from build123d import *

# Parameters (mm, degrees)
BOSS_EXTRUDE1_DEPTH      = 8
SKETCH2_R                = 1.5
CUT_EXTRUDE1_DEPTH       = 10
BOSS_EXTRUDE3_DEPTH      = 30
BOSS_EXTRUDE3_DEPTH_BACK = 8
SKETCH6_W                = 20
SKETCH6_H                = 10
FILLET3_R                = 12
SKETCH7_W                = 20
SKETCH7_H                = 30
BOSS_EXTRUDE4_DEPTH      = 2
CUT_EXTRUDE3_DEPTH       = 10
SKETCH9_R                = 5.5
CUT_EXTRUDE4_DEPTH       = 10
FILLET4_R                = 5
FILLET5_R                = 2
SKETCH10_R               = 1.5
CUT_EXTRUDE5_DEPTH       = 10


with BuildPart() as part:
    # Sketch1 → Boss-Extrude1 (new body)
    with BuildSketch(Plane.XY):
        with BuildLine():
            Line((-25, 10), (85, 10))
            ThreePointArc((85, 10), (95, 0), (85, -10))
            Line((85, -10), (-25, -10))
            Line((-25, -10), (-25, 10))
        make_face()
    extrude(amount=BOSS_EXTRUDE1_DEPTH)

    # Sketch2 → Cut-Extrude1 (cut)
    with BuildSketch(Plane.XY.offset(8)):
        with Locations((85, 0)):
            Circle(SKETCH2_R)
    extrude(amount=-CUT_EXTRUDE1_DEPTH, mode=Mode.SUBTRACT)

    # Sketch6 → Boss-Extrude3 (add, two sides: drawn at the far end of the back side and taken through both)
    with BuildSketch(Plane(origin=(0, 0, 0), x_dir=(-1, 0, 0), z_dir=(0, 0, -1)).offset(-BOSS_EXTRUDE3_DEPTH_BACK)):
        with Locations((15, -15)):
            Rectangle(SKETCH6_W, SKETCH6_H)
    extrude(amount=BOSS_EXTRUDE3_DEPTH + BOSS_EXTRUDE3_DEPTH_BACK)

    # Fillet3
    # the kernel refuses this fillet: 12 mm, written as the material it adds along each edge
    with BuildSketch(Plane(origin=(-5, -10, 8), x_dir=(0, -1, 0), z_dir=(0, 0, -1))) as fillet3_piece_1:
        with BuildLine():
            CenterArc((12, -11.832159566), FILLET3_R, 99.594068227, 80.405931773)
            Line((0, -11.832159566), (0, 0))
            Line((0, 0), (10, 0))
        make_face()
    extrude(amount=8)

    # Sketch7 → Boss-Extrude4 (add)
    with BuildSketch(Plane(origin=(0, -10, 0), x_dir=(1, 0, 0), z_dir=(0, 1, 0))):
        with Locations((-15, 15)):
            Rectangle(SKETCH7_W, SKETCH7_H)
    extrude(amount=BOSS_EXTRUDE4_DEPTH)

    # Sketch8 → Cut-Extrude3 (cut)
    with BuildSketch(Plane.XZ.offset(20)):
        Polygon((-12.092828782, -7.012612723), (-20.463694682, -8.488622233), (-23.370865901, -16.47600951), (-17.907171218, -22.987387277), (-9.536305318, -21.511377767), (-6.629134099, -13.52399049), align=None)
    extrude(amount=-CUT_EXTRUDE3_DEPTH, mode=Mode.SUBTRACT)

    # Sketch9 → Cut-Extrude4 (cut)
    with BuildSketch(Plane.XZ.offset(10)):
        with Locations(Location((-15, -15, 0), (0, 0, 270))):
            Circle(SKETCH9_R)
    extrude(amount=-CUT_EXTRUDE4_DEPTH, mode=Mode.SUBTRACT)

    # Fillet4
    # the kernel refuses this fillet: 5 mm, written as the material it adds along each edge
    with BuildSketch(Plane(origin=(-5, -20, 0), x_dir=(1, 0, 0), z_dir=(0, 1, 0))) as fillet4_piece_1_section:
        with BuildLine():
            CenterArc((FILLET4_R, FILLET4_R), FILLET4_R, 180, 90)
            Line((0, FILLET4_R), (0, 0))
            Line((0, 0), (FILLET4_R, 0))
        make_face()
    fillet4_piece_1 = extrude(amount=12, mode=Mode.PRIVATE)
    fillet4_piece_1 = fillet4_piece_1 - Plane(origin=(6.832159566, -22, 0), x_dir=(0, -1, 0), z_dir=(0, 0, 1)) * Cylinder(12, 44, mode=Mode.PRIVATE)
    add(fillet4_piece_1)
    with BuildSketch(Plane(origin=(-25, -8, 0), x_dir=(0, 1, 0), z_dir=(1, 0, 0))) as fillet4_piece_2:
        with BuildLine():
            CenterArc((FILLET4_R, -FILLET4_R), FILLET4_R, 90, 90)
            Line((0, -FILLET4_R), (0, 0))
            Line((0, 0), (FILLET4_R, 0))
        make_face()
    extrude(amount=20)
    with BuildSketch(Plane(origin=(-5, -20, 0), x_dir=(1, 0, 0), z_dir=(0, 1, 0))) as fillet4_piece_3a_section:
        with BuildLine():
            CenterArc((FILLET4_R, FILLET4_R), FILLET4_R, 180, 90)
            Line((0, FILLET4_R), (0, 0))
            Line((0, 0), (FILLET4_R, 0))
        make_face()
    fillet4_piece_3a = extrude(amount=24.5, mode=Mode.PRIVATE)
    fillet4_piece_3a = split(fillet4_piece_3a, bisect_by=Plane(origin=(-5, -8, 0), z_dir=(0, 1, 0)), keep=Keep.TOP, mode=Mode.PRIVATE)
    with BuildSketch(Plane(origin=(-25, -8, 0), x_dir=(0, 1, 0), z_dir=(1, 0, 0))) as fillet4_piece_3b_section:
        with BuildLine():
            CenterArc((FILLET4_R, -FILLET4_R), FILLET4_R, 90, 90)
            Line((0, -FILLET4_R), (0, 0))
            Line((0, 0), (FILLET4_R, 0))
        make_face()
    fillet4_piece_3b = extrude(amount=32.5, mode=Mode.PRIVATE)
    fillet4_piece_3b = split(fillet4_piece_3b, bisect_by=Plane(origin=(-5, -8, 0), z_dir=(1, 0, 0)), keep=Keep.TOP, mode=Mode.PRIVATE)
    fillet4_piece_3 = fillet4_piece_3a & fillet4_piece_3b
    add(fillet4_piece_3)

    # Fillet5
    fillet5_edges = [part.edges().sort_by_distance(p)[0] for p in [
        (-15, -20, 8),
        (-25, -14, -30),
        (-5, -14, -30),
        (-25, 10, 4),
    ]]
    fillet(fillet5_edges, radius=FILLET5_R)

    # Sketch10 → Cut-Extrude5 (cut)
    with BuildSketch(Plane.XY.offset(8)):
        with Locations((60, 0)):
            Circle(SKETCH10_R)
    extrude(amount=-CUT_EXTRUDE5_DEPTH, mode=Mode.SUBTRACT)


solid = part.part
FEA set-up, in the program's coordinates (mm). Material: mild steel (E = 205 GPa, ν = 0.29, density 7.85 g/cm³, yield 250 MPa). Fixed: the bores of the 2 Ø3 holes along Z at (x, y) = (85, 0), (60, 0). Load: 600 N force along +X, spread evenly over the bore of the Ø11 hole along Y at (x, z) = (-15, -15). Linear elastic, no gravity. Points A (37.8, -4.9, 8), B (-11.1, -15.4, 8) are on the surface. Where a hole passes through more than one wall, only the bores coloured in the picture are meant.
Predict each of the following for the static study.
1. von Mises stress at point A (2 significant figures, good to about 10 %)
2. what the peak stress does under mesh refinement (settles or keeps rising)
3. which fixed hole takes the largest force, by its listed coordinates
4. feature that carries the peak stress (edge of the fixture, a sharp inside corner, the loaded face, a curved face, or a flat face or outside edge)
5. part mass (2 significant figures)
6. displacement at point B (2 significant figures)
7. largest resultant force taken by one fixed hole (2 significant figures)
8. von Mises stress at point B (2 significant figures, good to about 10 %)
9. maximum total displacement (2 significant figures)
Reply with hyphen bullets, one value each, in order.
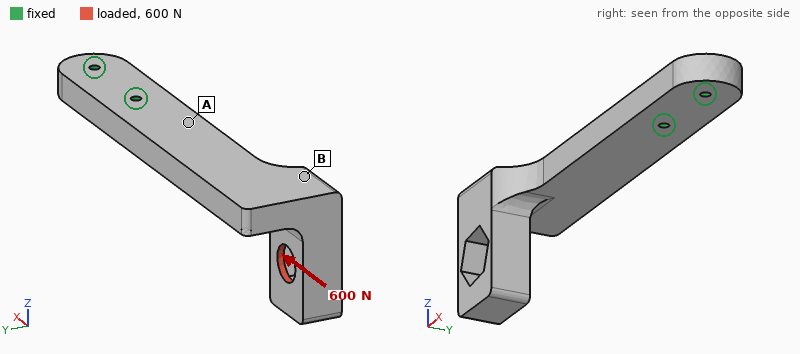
- 45 MPa
- keeps rising
- (60, 0)
- edge of the fixture
- 200 g
- 0.17 mm
- 560 N
- 14 MPa
- 0.29 mm
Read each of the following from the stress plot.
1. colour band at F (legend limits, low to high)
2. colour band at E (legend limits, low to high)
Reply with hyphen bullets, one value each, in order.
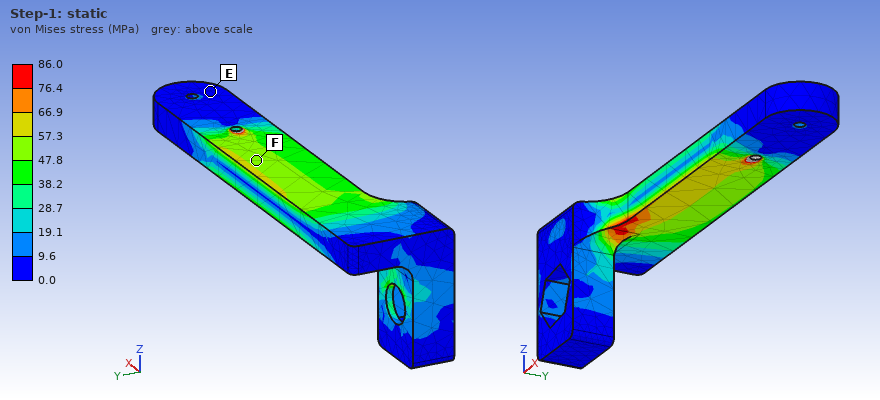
- 47.8 to 57.3 MPa
- 0.0 to 9.6 MPa
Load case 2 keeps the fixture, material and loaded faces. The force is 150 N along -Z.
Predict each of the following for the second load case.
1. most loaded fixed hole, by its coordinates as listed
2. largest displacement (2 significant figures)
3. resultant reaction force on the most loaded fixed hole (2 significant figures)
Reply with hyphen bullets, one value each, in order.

- (60, 0)
- 0.18 mm
- 310 N
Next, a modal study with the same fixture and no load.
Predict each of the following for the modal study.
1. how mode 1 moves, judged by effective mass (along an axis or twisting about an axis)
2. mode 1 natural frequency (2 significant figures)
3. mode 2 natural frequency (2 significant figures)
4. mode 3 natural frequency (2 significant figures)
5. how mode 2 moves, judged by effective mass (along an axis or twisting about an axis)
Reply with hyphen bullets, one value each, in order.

- along Z
- 540 Hz
- 1100 Hz
- 2100 Hz
- along Y
